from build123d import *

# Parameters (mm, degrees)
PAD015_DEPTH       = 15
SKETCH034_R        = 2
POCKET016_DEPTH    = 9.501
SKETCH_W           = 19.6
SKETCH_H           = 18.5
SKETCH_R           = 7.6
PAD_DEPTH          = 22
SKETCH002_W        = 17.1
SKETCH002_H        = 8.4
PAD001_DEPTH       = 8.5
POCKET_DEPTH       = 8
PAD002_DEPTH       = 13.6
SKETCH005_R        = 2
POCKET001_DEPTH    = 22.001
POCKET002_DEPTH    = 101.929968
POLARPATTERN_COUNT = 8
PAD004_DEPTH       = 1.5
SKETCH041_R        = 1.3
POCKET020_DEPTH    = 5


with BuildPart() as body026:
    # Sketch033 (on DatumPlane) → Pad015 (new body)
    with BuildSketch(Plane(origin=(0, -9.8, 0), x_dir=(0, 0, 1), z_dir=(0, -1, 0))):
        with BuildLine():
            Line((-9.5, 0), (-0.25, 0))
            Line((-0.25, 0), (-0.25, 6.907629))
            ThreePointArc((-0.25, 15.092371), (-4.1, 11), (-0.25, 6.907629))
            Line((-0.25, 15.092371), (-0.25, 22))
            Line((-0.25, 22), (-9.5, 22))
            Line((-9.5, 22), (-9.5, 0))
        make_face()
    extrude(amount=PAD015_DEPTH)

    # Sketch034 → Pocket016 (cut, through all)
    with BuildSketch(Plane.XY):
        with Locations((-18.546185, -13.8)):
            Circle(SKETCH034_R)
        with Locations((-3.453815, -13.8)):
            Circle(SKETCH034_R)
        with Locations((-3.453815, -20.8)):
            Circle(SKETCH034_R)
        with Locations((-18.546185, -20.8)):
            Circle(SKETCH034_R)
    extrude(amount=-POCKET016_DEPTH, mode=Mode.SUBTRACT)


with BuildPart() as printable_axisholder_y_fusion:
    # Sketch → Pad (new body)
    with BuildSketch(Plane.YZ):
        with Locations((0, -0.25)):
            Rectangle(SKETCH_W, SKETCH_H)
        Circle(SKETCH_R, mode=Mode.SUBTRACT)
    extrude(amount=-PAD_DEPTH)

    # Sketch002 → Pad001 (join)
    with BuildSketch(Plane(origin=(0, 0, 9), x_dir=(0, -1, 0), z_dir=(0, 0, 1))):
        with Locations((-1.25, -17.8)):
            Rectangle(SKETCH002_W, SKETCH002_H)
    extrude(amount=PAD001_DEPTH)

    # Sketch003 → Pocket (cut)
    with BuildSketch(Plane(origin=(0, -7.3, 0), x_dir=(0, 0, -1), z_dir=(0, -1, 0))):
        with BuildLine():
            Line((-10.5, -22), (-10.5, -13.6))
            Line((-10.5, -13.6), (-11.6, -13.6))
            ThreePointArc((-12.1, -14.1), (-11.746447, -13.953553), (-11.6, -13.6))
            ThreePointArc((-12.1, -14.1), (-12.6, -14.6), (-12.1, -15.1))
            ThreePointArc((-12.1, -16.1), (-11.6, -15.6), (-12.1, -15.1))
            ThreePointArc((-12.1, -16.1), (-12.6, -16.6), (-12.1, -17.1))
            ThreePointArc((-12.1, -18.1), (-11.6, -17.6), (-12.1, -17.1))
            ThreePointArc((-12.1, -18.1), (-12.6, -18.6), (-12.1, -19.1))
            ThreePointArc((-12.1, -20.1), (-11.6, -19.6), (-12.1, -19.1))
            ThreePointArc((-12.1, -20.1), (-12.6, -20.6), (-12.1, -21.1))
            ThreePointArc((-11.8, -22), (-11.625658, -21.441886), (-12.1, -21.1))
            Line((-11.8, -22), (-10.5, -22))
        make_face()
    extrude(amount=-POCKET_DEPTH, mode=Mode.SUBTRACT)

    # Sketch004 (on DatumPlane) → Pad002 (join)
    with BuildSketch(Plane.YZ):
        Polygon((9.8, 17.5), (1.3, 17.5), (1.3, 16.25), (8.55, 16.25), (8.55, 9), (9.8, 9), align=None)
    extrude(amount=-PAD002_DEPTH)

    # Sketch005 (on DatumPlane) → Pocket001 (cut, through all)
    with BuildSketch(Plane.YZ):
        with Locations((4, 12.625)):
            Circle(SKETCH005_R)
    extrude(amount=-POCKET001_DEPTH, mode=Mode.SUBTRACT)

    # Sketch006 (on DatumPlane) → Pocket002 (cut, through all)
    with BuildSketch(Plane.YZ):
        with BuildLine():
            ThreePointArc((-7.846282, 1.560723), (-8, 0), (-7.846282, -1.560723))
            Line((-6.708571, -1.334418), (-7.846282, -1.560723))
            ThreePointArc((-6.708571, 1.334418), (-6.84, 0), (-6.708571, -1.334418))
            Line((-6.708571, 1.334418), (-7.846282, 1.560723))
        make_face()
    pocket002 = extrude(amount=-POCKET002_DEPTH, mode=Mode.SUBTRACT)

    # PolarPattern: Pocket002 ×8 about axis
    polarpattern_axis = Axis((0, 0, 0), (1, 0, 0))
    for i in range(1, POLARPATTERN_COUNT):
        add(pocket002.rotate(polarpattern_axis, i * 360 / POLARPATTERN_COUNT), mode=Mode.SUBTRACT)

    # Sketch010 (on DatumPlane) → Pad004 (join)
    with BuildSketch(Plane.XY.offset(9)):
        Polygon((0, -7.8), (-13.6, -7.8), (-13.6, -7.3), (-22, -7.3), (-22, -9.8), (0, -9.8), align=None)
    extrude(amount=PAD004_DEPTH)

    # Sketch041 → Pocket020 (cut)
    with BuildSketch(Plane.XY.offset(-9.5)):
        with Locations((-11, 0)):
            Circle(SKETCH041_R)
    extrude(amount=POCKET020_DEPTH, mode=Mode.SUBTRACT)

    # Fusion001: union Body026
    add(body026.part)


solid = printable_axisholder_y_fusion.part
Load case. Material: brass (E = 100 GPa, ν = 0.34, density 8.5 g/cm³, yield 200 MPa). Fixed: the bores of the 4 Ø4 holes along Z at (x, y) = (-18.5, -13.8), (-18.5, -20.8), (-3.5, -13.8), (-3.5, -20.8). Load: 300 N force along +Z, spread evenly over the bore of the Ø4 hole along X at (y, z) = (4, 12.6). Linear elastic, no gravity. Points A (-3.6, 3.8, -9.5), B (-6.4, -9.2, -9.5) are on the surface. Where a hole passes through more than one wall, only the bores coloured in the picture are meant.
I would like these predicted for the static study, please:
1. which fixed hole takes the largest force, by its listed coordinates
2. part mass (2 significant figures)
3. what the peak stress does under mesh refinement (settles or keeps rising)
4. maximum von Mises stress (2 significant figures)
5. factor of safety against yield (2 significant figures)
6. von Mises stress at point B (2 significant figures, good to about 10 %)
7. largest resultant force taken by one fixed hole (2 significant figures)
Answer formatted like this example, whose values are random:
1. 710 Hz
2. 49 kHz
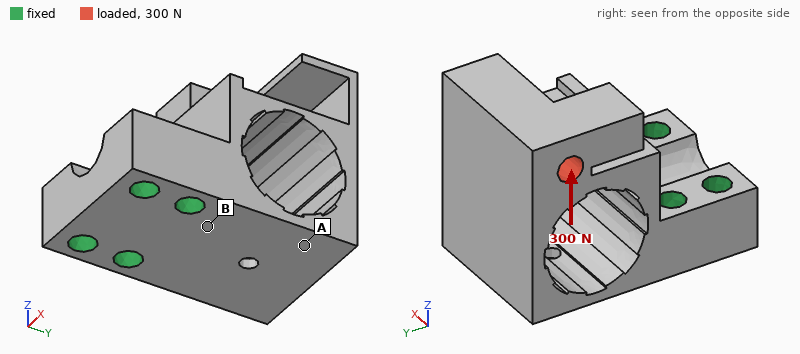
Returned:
1. (-18.5, -13.8)
2. 62 g
3. settles
4. 92 MPa
5. 2.2
6. 18 MPa
7. 290 N
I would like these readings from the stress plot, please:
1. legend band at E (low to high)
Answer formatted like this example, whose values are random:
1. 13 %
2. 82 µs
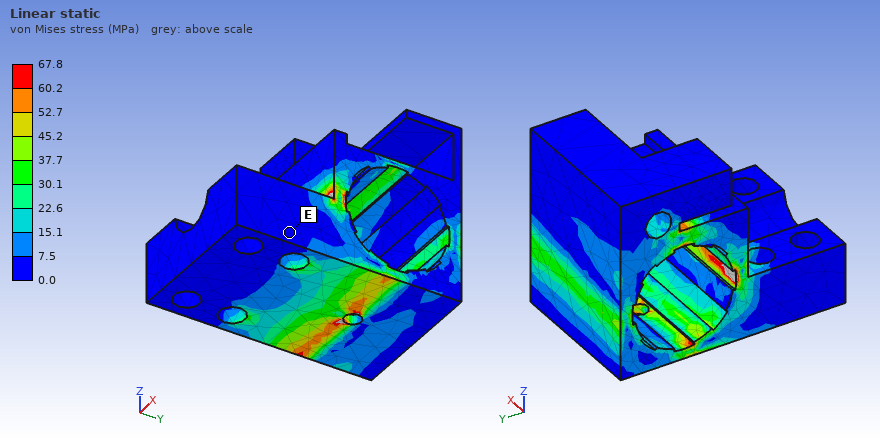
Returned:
1. 0.0 to 7.5 MPa
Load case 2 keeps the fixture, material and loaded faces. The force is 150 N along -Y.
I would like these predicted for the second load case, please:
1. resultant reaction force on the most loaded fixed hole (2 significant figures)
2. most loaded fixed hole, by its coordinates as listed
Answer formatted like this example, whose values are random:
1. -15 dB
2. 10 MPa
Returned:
1. 140 N
2. (-18.5, -13.8)
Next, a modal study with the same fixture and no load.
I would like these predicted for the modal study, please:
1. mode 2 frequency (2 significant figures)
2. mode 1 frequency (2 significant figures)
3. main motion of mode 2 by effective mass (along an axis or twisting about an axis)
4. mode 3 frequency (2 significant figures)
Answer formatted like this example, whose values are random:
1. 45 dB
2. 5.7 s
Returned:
1. 4600 Hz
2. 2100 Hz
3. along X
4. 7800 Hz
